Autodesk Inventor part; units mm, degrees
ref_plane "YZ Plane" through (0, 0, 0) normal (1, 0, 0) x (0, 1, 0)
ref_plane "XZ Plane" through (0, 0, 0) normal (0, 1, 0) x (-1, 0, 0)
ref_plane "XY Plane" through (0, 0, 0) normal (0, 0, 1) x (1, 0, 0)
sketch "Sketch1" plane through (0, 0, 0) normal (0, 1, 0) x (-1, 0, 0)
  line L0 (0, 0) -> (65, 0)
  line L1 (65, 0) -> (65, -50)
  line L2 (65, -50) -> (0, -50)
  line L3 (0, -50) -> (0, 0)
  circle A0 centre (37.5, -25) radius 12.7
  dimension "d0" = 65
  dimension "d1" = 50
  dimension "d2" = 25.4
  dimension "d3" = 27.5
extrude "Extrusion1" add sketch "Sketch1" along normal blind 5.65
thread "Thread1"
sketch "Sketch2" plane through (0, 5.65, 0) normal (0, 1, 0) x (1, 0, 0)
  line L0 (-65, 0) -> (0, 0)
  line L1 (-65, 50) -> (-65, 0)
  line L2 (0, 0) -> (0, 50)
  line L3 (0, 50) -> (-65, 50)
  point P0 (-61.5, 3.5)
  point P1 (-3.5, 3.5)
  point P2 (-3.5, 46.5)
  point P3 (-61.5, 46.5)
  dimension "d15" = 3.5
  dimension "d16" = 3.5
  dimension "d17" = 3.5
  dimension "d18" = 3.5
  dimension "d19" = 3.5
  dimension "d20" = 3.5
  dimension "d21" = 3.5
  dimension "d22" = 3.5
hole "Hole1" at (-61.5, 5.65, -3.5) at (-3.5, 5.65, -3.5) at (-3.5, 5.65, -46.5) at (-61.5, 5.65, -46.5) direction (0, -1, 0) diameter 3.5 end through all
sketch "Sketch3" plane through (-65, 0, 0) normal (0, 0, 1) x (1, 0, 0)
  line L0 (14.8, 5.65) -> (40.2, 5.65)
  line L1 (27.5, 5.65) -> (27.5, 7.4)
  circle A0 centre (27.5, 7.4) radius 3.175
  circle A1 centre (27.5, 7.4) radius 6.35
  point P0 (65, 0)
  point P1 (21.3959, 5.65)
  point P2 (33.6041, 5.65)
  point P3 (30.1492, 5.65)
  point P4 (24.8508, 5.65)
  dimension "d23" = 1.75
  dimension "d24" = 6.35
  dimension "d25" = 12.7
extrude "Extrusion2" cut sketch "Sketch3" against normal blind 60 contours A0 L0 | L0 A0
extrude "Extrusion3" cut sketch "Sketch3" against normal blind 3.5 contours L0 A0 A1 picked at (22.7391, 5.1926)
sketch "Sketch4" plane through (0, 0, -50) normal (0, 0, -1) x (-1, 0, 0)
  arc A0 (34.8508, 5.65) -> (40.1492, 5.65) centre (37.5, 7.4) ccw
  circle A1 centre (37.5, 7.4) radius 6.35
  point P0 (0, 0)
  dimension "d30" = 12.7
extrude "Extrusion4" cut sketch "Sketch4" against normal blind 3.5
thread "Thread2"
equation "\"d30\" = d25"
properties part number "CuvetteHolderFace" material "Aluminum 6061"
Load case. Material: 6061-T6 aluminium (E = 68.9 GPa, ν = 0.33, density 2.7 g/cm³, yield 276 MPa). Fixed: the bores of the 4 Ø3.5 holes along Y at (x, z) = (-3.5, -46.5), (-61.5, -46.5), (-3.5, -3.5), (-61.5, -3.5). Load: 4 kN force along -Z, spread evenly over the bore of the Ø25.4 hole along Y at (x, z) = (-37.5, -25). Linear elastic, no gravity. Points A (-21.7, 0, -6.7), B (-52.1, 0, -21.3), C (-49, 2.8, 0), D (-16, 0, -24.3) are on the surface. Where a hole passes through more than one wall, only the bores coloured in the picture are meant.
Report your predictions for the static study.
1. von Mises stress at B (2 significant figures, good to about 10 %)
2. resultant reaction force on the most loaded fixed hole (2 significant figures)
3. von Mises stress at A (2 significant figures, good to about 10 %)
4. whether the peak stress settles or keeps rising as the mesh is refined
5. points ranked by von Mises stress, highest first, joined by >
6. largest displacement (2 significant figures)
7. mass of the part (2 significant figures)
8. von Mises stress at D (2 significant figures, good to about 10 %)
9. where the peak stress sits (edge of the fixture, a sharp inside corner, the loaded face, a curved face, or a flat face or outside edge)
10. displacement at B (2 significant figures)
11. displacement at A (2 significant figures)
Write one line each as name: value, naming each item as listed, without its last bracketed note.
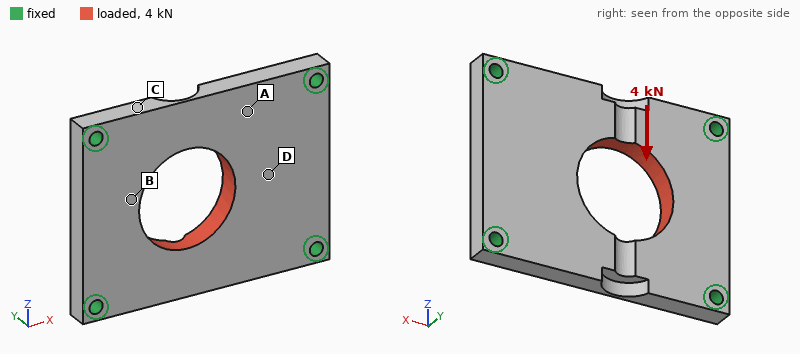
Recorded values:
von Mises stress at B: 23 MPa
resultant reaction force on the most loaded fixed hole: 1.2 kN
von Mises stress at A: 9.1 MPa
whether the peak stress settles or keeps rising as the mesh is refined: keeps rising
points ranked by von Mises stress, highest first, joined by >: B > D > A > C
largest displacement: 13 µm
mass of the part: 40 g
von Mises stress at D: 17 MPa
where the peak stress sits: edge of the fixture
displacement at B: 5.4 µm
displacement at A: 7.6 µm
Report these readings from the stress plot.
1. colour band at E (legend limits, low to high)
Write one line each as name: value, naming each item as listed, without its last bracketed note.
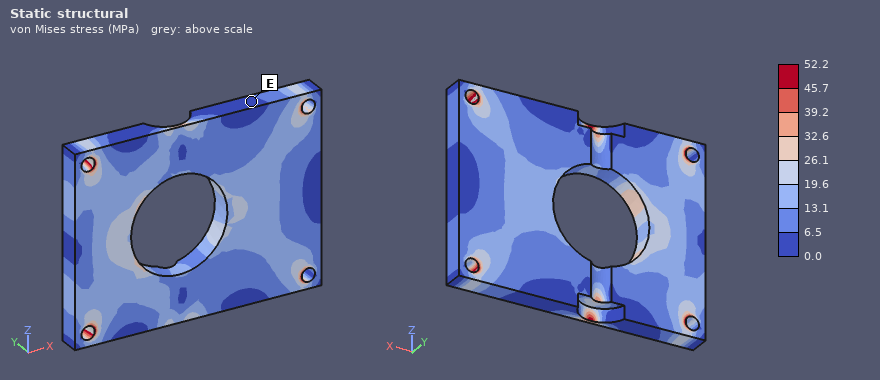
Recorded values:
colour band at E: 0.0 to 6.5 MPa
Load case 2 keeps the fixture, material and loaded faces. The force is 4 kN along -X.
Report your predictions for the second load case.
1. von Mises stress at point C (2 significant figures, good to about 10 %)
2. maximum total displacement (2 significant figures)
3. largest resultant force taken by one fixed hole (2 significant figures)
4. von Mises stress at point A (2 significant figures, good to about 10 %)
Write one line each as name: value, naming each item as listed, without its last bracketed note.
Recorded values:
von Mises stress at point C: 10 MPa
maximum total displacement: 9.3 µm
largest resultant force taken by one fixed hole: 1.2 kN
von Mises stress at point A: 9.0 MPa
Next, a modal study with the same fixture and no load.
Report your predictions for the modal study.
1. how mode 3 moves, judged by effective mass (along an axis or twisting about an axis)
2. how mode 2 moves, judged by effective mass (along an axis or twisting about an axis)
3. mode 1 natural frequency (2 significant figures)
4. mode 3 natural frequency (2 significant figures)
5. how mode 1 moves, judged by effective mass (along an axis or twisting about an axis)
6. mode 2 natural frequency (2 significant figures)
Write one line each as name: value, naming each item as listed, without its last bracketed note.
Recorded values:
how mode 3 moves, judged by effective mass: twisting about Z
how mode 2 moves, judged by effective mass: twisting about X
mode 1 natural frequency: 6600 Hz
mode 3 natural frequency: 13 kHz
how mode 1 moves, judged by effective mass: along Y
mode 2 natural frequency: 9600 Hz
